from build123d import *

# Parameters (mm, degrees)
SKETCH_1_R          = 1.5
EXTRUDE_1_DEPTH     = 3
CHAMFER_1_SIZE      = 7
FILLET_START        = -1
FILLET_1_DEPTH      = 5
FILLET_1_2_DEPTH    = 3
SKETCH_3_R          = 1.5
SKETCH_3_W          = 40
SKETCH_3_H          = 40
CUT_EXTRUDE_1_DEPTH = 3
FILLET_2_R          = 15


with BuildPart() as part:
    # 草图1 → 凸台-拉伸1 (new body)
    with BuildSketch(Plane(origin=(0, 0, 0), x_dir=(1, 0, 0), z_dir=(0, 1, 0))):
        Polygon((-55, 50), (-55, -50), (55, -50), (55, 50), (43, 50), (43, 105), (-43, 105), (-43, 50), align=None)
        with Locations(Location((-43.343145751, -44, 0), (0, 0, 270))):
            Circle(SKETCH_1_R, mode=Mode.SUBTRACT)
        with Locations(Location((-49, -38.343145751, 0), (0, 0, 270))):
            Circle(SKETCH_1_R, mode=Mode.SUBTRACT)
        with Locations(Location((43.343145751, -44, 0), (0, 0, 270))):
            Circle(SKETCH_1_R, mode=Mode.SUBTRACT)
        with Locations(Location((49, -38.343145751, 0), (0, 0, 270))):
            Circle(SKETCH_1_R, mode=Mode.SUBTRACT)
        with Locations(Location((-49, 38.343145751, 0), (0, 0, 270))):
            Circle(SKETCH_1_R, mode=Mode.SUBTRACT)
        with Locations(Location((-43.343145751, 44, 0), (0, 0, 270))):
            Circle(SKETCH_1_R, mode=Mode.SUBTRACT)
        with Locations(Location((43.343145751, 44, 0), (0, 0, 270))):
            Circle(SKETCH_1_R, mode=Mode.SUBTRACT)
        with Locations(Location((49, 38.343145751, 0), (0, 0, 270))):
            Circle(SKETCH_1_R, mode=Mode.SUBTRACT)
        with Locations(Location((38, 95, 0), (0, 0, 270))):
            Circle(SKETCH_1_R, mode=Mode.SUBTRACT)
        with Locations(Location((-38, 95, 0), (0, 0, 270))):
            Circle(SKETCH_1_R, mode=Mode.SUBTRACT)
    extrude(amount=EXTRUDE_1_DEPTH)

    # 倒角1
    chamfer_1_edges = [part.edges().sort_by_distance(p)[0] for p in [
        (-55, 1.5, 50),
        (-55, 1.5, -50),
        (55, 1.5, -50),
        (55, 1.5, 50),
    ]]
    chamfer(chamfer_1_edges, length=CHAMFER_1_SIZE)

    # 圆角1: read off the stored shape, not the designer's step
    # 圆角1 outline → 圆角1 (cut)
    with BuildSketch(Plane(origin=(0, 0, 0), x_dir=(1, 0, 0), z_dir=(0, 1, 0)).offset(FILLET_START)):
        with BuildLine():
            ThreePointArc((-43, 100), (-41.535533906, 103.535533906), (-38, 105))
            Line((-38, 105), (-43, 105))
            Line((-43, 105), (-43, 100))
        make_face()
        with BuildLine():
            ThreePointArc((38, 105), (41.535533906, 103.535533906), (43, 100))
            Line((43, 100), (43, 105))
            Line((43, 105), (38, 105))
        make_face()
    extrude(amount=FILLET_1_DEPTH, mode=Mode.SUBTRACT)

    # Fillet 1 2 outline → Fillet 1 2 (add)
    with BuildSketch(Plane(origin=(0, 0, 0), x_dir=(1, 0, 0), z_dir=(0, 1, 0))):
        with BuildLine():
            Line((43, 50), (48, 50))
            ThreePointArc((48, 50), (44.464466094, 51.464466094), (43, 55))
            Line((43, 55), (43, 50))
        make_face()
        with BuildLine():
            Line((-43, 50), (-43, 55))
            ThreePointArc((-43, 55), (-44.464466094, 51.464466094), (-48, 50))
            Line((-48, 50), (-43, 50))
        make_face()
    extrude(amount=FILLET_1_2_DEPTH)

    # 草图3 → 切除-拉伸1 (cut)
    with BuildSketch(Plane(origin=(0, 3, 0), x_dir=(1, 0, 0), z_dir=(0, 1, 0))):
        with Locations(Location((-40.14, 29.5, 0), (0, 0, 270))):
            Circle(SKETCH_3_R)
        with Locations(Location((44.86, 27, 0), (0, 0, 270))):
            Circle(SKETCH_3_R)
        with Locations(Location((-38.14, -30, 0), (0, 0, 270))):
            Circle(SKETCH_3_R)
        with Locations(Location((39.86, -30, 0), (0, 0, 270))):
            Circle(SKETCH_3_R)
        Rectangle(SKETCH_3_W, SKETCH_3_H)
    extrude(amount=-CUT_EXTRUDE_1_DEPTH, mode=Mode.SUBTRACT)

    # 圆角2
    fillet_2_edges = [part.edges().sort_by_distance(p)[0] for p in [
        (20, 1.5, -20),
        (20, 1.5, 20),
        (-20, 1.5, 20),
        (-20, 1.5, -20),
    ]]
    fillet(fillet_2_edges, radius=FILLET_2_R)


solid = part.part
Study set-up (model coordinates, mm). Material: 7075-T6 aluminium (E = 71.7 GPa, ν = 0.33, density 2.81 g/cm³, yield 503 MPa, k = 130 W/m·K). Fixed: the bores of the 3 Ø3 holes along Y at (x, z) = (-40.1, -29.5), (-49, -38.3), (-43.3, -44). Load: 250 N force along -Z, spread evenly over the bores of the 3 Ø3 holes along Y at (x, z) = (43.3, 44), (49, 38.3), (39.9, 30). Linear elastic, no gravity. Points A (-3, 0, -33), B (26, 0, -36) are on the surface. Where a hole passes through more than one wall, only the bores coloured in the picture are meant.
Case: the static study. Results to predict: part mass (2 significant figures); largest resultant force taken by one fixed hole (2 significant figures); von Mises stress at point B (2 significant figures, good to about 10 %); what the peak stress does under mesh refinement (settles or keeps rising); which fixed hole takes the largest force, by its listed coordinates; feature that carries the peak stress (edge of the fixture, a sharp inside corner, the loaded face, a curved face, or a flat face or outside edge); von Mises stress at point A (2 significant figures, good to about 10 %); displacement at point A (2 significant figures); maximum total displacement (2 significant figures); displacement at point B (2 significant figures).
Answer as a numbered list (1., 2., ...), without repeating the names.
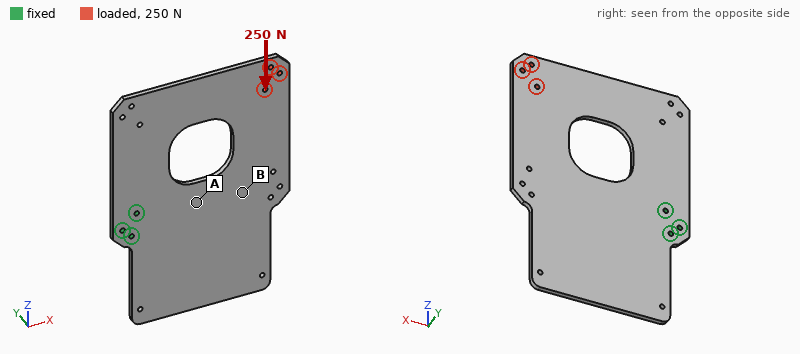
1. 120 g
2. 1.2 kN
3. 2.4 MPa
4. keeps rising
5. (-40.1, -29.5)
6. edge of the fixture
7. 4.6 MPa
8. 27 µm
9. 90 µm
10. 48 µm
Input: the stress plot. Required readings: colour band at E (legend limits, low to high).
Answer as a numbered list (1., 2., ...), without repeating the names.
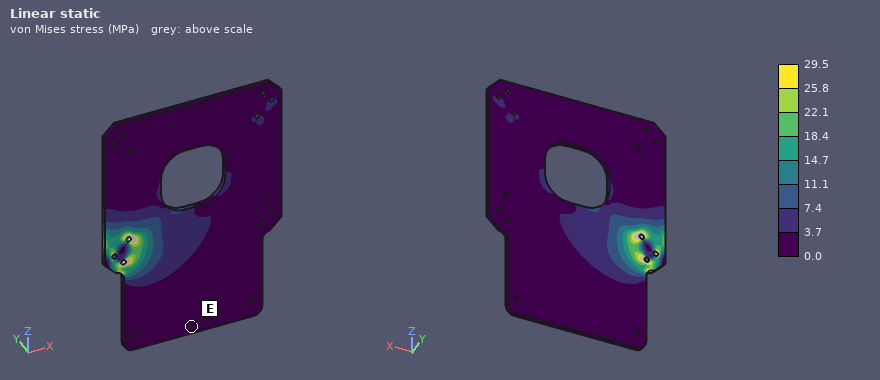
1. 0.0 to 3.7 MPa
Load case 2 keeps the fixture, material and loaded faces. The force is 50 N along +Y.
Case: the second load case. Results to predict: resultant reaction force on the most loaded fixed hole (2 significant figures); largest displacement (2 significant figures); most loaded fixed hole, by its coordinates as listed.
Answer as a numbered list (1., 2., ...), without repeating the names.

1. 270 N
2. 2.2 mm
3. (-40.1, -29.5)
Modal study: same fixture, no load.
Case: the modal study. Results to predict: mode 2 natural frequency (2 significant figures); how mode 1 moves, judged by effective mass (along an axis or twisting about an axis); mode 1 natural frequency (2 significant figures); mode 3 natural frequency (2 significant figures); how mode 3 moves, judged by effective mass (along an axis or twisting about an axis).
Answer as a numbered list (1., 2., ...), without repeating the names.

1. 230 Hz
2. along Y
3. 180 Hz
4. 470 Hz
5. along Y
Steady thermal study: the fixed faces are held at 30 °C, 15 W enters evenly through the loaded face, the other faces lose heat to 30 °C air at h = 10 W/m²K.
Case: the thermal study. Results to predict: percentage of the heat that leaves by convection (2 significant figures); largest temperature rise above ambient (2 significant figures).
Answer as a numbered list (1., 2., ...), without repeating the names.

1. 41 %
2. 66 K
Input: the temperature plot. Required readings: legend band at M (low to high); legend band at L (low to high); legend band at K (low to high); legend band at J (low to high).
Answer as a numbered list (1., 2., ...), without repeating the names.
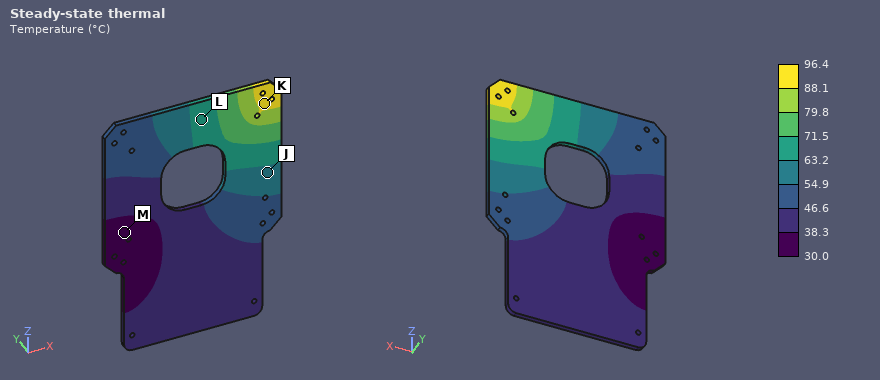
1. 30.0 to 38.3 °C
2. 63.2 to 71.5 °C
3. 88.1 to 96.4 °C
4. 54.9 to 63.2 °C
